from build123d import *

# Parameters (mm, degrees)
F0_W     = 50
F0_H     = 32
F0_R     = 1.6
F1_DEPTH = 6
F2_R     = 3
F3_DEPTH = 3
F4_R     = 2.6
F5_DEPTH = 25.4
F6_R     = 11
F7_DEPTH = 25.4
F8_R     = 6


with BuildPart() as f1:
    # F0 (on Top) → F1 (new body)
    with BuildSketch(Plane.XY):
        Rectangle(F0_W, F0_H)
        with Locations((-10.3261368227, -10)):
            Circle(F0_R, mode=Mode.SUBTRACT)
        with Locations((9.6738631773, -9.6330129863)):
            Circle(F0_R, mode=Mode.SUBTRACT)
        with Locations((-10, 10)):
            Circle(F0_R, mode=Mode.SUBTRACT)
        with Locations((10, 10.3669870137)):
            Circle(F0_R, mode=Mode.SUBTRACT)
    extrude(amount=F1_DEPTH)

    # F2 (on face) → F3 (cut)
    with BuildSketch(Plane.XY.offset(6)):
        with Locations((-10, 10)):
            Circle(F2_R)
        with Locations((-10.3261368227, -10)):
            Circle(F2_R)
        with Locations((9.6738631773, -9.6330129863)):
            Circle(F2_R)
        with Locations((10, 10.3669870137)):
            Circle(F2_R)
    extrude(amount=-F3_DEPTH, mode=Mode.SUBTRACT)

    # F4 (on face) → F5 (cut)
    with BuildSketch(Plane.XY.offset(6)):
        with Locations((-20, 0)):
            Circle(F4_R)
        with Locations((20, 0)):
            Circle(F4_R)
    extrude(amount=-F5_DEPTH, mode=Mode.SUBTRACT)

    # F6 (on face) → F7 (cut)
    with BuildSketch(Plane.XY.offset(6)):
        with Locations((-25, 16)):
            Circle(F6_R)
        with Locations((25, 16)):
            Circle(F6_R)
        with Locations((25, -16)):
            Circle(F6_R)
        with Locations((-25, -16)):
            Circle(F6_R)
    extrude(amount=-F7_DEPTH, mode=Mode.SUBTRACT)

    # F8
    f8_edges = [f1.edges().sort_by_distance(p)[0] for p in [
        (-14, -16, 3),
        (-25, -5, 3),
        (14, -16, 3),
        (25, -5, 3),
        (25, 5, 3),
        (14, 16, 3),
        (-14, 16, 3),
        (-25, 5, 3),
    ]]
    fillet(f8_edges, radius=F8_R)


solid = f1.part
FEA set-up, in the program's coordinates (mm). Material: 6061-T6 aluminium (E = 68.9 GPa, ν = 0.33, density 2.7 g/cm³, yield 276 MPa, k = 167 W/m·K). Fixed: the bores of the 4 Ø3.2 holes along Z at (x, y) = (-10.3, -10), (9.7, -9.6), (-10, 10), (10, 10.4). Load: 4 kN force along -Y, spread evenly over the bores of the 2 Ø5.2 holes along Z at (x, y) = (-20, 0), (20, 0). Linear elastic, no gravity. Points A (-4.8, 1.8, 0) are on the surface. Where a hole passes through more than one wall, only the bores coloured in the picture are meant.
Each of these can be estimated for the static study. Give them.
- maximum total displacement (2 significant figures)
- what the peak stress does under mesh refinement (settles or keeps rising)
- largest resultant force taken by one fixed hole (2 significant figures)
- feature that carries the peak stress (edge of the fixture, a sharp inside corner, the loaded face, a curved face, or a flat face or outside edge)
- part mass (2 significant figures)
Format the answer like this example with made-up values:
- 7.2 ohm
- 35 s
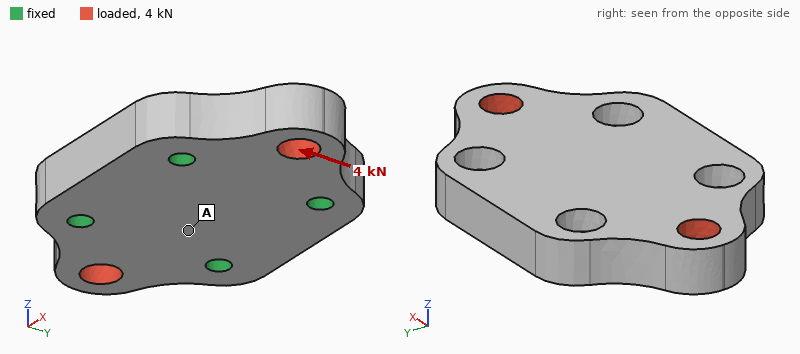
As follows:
- 18 µm
- keeps rising
- 1.2 kN
- edge of the fixture
- 17 g
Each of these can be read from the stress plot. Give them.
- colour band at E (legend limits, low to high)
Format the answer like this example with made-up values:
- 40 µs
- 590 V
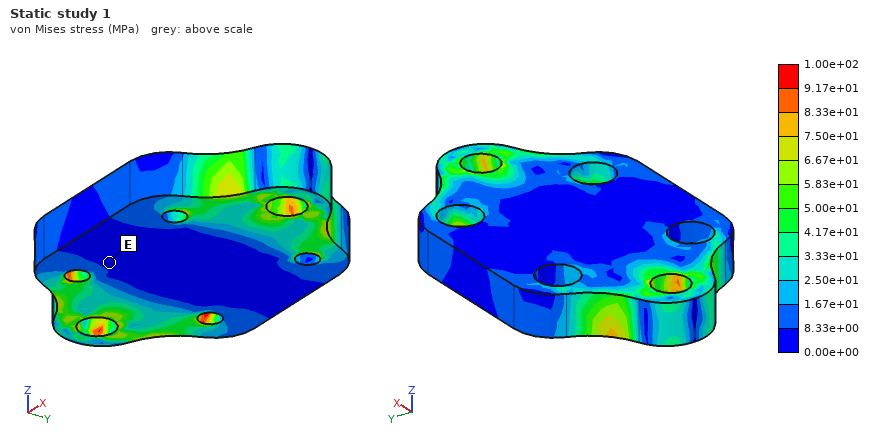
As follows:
- 0.00e+00 to 8.33e+00 MPa
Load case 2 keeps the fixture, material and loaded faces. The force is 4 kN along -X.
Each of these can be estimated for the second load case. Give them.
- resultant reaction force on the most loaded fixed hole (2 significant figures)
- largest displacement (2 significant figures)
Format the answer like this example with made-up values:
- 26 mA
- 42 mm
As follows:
- 1.1 kN
- 13 µm
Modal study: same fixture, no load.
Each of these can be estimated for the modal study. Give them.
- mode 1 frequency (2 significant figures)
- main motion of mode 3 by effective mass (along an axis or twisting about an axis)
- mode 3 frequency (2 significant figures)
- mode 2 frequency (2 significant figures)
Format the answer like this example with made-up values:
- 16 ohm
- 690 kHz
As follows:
- 20 kHz
- along Z
- 35 kHz
- 20 kHz
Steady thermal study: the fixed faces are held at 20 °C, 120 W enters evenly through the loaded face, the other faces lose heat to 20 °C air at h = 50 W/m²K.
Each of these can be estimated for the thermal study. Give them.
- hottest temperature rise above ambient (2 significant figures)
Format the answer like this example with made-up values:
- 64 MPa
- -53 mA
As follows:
- 64 K
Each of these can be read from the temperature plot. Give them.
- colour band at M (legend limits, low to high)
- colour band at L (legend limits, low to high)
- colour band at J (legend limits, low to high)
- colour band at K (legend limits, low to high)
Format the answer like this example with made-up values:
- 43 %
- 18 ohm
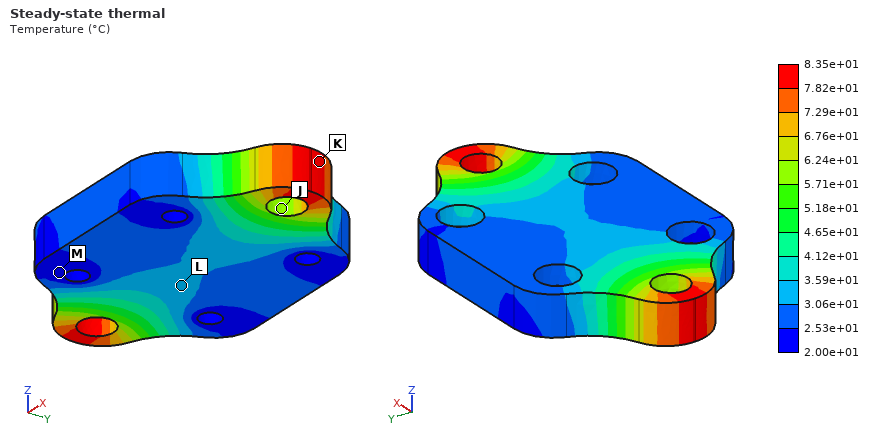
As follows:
- 2.00e+01 to 2.53e+01 °C
- 3.06e+01 to 3.59e+01 °C
- 5.71e+01 to 6.24e+01 °C
- 7.82e+01 to 8.35e+01 °C
